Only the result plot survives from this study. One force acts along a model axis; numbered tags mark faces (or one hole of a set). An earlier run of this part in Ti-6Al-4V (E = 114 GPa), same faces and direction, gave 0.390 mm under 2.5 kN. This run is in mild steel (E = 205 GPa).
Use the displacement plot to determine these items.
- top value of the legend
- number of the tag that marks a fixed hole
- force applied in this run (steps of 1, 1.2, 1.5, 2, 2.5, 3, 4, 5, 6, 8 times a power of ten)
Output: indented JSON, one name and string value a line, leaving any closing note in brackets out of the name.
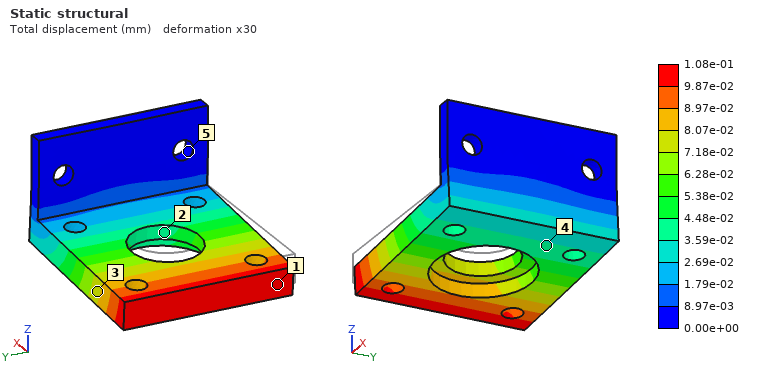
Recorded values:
{
  "top value of the legend": "1.08e-01 mm",
  "number of the tag that marks a fixed hole": "5",
  "force applied in this run": "1.2 kN"
}
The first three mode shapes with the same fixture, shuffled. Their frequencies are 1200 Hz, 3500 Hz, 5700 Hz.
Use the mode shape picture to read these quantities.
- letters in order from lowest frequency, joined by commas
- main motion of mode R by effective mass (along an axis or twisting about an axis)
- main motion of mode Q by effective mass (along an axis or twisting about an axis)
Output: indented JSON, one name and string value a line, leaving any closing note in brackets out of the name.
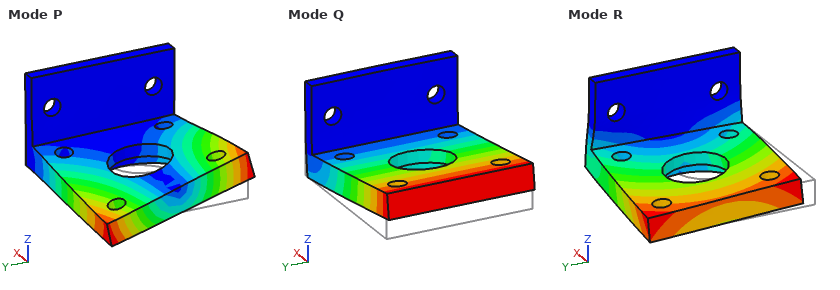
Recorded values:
{
  "letters in order from lowest frequency, joined by commas": "Q, R, P",
  "main motion of mode R by effective mass": "along Y",
  "main motion of mode Q by effective mass": "along Z"
}
